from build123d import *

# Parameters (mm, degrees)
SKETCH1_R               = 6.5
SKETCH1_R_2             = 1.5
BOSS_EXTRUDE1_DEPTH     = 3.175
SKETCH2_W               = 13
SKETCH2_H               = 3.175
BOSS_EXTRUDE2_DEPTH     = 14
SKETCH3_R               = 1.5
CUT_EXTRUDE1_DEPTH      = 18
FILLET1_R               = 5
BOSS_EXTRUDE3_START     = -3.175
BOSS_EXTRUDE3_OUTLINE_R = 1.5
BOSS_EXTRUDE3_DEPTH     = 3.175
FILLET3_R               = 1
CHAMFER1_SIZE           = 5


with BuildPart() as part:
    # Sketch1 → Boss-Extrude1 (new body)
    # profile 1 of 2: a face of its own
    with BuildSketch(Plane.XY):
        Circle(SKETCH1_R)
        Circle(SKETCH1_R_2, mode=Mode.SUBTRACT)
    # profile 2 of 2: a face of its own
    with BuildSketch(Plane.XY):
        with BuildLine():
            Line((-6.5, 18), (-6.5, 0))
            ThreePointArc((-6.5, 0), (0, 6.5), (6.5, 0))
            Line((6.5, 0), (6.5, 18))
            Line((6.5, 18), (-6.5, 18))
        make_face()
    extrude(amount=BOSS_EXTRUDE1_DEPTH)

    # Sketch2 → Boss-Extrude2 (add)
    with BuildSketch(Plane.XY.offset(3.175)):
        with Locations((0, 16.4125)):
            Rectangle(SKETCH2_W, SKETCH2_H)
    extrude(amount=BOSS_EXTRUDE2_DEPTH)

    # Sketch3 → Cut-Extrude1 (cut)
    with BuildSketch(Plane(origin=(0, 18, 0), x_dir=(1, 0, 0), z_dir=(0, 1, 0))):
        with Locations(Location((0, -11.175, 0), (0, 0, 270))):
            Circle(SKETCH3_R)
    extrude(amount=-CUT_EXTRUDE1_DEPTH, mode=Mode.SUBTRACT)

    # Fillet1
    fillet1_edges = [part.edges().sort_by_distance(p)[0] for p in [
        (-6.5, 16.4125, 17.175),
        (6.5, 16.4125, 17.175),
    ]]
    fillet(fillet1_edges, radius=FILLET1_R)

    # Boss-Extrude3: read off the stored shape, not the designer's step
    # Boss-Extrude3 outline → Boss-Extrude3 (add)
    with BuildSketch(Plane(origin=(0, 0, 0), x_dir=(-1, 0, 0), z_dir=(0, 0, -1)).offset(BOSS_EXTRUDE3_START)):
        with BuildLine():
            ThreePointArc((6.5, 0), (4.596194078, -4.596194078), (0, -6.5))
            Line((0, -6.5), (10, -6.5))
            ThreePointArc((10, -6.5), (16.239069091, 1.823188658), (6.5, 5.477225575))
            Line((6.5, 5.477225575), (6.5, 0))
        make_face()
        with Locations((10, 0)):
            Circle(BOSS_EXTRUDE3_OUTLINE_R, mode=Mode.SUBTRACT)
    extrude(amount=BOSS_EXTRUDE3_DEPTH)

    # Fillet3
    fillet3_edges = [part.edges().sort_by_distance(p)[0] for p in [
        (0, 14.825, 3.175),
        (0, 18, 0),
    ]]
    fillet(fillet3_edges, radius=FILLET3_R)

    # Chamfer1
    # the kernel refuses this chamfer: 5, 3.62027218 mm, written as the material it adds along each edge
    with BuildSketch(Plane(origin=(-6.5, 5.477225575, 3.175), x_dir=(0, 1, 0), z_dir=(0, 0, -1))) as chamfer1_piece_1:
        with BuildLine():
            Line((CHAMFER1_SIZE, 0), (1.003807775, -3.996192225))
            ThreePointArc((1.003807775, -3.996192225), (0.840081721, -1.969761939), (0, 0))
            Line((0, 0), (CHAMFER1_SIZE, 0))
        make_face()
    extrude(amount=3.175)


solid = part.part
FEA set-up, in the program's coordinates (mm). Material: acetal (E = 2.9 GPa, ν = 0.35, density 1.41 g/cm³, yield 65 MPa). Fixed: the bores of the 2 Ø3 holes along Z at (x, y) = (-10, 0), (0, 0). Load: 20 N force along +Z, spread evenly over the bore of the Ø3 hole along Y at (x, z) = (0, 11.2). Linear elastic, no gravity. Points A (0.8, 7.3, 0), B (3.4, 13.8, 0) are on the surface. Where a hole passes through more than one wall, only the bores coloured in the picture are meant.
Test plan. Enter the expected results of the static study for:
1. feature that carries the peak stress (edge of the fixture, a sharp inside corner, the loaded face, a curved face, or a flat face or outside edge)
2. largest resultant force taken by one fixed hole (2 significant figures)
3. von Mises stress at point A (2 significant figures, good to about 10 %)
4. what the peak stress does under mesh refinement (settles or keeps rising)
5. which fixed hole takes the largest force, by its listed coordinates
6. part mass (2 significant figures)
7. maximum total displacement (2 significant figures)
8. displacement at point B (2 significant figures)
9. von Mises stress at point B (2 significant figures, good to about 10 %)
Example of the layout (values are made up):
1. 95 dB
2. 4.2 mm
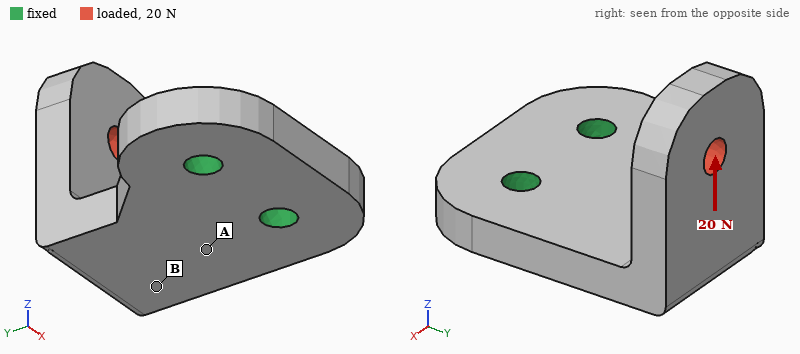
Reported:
1. edge of the fixture
2. 18 N
3. 6.4 MPa
4. keeps rising
5. (0, 0)
6. 2.6 g
7. 0.42 mm
8. 0.18 mm
9. 2.2 MPa
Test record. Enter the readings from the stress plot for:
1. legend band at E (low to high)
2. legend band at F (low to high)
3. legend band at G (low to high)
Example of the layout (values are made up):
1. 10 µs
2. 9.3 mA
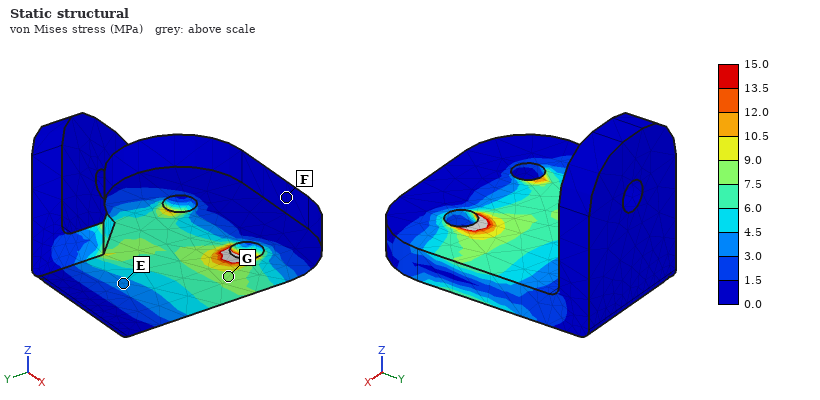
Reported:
1. 3.0 to 4.5 MPa
2. 0.0 to 1.5 MPa
3. 7.5 to 9.0 MPa
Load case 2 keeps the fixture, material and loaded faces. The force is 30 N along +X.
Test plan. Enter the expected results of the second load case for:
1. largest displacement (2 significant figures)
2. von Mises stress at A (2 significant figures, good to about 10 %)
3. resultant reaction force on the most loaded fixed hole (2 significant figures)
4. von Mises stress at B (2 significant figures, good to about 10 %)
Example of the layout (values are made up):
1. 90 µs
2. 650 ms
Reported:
1. 0.39 mm
2. 8.2 MPa
3. 49 N
4. 6.6 MPa
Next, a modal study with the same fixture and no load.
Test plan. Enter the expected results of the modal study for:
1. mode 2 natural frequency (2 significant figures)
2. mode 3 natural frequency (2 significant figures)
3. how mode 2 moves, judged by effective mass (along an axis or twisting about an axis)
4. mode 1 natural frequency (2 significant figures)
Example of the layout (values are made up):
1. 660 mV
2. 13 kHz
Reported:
1. 2000 Hz
2. 3200 Hz
3. along X
4. 1200 Hz
